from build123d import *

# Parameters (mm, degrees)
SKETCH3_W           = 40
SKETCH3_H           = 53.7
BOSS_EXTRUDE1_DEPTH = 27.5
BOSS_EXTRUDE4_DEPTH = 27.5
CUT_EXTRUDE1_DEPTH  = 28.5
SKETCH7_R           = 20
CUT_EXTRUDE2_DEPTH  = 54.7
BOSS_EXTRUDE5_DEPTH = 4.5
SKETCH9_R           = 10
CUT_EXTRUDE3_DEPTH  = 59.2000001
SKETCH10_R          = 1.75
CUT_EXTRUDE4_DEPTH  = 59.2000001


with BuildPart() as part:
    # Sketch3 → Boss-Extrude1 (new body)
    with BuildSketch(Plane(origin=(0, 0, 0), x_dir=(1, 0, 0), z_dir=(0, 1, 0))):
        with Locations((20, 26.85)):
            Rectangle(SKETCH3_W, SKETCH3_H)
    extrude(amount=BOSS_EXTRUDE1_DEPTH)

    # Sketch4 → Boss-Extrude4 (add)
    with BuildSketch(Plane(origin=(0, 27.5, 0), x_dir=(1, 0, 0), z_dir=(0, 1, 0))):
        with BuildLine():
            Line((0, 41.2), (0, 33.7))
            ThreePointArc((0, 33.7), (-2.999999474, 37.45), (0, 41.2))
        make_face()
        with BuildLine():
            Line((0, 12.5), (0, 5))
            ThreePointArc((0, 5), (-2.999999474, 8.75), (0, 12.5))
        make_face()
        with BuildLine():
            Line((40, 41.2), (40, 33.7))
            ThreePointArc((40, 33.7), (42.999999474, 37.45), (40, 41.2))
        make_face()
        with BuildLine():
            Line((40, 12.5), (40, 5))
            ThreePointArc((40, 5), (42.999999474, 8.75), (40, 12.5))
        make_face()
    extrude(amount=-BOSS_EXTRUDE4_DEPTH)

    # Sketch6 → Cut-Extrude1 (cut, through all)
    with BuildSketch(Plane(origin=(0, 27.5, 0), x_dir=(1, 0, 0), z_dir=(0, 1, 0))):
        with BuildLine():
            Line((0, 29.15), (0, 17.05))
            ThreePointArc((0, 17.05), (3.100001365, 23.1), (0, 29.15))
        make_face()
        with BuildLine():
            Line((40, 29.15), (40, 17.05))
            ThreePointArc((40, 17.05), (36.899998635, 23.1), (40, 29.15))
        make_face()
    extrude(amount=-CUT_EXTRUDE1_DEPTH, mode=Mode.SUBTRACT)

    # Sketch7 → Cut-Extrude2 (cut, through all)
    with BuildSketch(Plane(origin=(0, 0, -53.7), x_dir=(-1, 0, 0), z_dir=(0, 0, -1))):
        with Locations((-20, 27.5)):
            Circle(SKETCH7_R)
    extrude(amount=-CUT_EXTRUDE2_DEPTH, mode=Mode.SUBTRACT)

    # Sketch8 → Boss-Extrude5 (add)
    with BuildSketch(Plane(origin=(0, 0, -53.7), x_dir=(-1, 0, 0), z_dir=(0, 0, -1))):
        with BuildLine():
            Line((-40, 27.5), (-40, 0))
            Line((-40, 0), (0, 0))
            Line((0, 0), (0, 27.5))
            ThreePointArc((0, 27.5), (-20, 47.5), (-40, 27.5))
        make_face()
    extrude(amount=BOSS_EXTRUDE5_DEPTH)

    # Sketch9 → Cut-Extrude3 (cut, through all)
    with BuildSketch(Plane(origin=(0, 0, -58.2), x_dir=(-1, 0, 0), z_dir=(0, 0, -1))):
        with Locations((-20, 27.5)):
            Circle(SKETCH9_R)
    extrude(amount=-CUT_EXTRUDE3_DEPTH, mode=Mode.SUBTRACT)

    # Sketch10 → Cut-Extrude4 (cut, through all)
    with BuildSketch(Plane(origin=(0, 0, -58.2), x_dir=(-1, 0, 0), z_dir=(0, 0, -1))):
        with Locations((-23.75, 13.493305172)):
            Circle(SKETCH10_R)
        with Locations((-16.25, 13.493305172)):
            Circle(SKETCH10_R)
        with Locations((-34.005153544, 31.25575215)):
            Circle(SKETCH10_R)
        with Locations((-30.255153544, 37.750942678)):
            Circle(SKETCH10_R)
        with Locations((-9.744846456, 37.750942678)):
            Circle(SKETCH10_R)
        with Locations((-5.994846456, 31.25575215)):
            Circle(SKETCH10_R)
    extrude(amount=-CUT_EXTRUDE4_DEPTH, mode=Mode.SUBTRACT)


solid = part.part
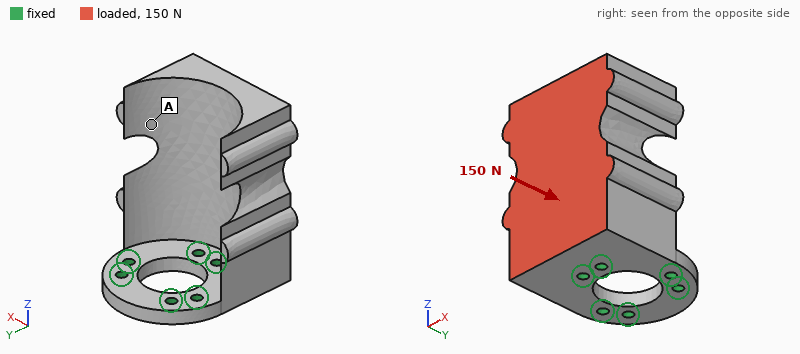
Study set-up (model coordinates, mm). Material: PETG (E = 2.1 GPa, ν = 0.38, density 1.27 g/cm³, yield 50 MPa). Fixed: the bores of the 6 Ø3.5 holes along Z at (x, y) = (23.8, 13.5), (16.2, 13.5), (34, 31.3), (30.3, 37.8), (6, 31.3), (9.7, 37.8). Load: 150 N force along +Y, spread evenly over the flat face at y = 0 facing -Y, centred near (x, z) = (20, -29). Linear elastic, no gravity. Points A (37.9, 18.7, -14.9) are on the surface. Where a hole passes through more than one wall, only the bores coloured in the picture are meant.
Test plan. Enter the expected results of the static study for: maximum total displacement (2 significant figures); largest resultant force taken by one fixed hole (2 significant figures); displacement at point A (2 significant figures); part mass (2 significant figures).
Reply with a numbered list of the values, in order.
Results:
1. 1.0 mm
2. 110 N
3. 0.73 mm
4. 41 g
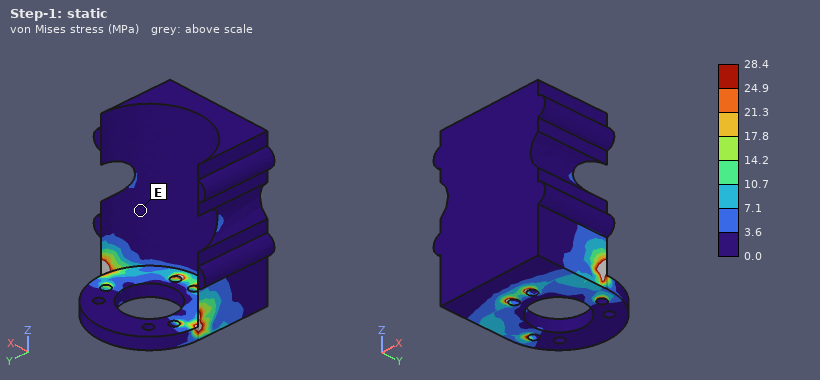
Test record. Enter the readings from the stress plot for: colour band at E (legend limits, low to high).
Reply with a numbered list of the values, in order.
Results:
1. 0.0 to 3.6 MPa
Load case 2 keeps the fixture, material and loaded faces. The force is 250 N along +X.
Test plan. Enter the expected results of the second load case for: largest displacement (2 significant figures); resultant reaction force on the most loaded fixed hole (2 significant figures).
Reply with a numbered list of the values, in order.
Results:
1. 0.98 mm
2. 270 N
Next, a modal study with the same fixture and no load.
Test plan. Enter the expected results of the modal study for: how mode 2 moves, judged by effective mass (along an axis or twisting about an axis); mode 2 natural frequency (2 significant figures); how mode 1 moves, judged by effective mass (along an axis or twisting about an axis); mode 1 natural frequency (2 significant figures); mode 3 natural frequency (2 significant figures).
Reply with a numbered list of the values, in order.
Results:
1. along X
2. 480 Hz
3. along Y
4. 390 Hz
5. 1200 Hz
